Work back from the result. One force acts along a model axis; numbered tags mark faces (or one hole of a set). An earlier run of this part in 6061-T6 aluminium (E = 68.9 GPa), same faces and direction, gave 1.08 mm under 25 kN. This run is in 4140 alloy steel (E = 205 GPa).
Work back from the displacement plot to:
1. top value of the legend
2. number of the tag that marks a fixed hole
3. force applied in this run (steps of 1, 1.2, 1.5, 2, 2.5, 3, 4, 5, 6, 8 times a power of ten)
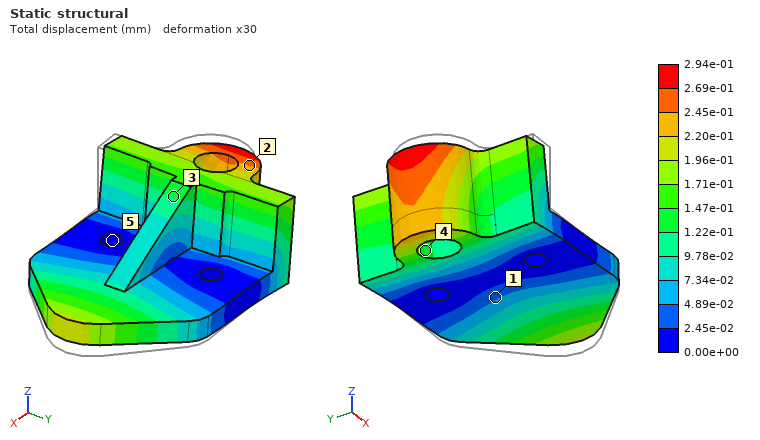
2.94e-01 mm
5
20 kN
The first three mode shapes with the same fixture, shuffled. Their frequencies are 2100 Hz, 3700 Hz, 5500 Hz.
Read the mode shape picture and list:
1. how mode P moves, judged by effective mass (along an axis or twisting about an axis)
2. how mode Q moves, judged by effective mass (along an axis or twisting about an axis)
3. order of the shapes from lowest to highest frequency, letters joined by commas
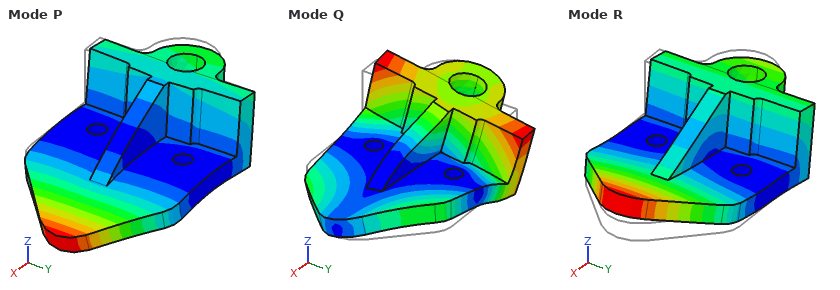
along Z
along Y
R, P, Q
